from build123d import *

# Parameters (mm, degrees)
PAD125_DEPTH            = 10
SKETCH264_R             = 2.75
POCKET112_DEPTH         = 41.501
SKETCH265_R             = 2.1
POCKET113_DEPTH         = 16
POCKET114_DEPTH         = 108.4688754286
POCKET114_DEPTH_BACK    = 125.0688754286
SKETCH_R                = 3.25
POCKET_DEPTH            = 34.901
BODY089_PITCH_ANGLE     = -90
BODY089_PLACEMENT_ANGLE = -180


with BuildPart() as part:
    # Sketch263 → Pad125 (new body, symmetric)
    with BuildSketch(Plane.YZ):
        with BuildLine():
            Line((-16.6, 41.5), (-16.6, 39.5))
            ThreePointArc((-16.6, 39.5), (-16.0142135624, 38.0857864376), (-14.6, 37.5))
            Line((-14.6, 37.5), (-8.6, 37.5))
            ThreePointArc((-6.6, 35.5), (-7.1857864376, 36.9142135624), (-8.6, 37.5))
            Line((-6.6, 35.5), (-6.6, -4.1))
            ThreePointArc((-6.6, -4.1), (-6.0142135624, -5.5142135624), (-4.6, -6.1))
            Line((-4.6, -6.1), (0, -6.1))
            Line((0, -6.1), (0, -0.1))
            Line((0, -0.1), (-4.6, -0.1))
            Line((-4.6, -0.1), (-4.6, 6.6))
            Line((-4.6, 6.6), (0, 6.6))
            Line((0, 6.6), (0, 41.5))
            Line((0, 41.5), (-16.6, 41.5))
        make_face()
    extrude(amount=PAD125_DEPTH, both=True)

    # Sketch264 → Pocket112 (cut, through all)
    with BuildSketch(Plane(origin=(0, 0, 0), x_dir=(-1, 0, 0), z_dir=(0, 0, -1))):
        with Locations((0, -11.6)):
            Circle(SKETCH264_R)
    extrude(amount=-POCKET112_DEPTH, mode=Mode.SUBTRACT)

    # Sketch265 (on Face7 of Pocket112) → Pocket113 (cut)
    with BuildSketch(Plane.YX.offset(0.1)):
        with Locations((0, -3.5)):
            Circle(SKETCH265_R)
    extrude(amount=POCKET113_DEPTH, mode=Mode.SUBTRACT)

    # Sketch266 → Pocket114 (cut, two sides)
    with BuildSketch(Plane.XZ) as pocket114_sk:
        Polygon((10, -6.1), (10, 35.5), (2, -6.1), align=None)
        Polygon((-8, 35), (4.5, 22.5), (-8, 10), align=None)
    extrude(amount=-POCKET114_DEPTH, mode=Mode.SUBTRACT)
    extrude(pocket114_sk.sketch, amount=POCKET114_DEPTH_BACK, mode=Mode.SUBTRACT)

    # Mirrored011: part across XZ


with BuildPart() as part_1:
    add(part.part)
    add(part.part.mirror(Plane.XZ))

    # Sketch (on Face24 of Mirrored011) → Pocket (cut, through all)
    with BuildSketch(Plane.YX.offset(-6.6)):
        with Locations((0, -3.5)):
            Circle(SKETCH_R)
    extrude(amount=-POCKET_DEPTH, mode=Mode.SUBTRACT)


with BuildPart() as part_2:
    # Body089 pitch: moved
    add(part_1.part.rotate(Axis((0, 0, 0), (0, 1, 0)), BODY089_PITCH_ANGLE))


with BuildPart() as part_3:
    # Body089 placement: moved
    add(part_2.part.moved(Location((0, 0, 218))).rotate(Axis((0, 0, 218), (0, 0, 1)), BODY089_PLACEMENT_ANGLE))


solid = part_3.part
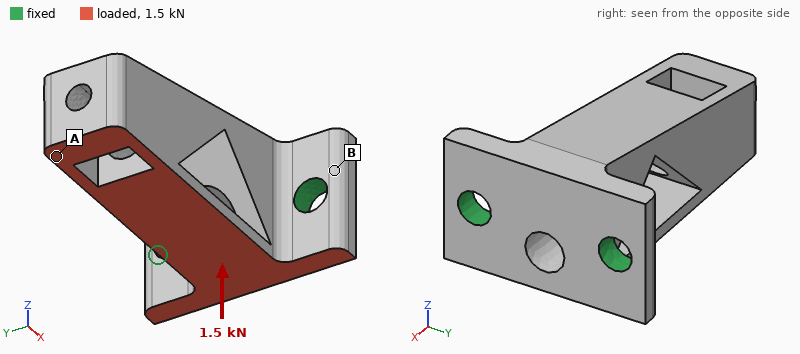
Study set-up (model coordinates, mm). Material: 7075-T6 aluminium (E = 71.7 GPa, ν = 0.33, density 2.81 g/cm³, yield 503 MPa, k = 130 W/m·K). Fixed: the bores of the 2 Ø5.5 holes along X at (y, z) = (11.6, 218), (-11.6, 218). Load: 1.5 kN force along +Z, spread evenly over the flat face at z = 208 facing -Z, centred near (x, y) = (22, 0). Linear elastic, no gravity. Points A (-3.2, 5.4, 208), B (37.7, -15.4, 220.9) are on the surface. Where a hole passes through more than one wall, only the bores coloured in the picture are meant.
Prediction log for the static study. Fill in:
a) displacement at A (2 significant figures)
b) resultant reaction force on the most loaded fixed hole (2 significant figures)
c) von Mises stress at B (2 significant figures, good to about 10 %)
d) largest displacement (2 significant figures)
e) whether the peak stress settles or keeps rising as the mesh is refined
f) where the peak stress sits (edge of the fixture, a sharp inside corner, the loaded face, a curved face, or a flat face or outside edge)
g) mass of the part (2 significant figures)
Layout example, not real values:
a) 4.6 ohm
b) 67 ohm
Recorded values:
a) 0.24 mm
b) 750 N
c) 58 MPa
d) 0.26 mm
e) keeps rising
f) edge of the fixture
g) 23 g
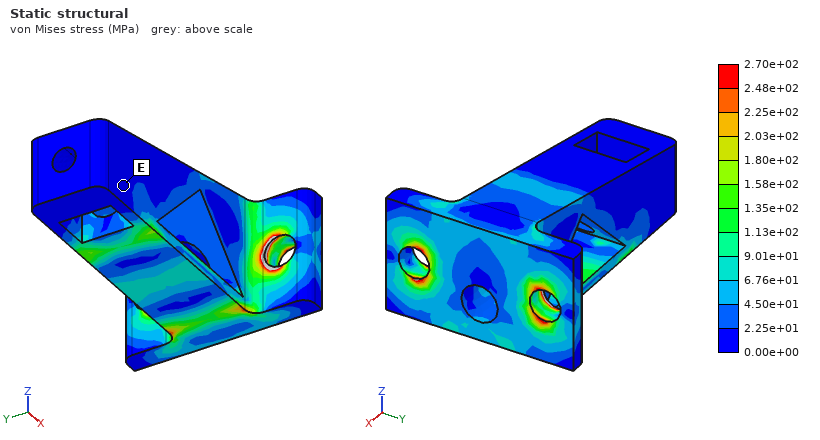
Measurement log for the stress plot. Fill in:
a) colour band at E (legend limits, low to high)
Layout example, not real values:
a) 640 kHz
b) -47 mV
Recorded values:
a) 0.00e+00 to 2.25e+01 MPa
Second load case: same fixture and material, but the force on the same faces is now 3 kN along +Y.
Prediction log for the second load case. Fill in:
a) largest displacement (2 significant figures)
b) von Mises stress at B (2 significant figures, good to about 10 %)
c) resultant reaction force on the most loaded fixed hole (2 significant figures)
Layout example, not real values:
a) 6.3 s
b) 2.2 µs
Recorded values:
a) 0.40 mm
b) 29 MPa
c) 3.5 kN
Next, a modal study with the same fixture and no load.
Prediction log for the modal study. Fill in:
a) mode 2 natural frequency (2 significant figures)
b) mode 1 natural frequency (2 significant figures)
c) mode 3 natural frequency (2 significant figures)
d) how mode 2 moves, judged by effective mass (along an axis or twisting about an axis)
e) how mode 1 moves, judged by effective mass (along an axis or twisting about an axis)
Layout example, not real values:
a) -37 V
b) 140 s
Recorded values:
a) 4200 Hz
b) 3300 Hz
c) 13 kHz
d) along Y
e) along Z
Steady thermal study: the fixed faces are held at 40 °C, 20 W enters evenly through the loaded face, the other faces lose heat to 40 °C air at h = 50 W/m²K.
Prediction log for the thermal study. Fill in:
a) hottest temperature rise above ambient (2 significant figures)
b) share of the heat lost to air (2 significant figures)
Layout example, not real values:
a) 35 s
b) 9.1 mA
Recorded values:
a) 29 K
b) 15 %
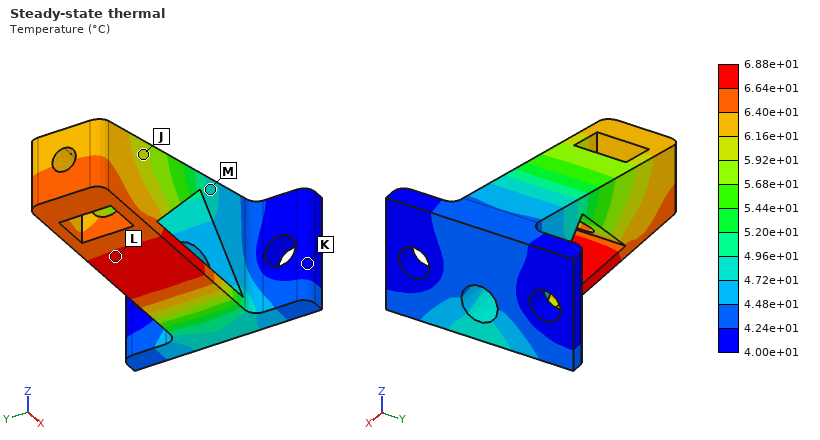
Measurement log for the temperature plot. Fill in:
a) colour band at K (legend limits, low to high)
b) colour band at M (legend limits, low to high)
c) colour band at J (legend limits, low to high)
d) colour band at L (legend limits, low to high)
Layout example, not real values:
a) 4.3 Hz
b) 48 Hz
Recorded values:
a) 4.00e+01 to 4.24e+01 °C
b) 4.72e+01 to 4.96e+01 °C
c) 5.92e+01 to 6.16e+01 °C
d) 6.64e+01 to 6.88e+01 °C
